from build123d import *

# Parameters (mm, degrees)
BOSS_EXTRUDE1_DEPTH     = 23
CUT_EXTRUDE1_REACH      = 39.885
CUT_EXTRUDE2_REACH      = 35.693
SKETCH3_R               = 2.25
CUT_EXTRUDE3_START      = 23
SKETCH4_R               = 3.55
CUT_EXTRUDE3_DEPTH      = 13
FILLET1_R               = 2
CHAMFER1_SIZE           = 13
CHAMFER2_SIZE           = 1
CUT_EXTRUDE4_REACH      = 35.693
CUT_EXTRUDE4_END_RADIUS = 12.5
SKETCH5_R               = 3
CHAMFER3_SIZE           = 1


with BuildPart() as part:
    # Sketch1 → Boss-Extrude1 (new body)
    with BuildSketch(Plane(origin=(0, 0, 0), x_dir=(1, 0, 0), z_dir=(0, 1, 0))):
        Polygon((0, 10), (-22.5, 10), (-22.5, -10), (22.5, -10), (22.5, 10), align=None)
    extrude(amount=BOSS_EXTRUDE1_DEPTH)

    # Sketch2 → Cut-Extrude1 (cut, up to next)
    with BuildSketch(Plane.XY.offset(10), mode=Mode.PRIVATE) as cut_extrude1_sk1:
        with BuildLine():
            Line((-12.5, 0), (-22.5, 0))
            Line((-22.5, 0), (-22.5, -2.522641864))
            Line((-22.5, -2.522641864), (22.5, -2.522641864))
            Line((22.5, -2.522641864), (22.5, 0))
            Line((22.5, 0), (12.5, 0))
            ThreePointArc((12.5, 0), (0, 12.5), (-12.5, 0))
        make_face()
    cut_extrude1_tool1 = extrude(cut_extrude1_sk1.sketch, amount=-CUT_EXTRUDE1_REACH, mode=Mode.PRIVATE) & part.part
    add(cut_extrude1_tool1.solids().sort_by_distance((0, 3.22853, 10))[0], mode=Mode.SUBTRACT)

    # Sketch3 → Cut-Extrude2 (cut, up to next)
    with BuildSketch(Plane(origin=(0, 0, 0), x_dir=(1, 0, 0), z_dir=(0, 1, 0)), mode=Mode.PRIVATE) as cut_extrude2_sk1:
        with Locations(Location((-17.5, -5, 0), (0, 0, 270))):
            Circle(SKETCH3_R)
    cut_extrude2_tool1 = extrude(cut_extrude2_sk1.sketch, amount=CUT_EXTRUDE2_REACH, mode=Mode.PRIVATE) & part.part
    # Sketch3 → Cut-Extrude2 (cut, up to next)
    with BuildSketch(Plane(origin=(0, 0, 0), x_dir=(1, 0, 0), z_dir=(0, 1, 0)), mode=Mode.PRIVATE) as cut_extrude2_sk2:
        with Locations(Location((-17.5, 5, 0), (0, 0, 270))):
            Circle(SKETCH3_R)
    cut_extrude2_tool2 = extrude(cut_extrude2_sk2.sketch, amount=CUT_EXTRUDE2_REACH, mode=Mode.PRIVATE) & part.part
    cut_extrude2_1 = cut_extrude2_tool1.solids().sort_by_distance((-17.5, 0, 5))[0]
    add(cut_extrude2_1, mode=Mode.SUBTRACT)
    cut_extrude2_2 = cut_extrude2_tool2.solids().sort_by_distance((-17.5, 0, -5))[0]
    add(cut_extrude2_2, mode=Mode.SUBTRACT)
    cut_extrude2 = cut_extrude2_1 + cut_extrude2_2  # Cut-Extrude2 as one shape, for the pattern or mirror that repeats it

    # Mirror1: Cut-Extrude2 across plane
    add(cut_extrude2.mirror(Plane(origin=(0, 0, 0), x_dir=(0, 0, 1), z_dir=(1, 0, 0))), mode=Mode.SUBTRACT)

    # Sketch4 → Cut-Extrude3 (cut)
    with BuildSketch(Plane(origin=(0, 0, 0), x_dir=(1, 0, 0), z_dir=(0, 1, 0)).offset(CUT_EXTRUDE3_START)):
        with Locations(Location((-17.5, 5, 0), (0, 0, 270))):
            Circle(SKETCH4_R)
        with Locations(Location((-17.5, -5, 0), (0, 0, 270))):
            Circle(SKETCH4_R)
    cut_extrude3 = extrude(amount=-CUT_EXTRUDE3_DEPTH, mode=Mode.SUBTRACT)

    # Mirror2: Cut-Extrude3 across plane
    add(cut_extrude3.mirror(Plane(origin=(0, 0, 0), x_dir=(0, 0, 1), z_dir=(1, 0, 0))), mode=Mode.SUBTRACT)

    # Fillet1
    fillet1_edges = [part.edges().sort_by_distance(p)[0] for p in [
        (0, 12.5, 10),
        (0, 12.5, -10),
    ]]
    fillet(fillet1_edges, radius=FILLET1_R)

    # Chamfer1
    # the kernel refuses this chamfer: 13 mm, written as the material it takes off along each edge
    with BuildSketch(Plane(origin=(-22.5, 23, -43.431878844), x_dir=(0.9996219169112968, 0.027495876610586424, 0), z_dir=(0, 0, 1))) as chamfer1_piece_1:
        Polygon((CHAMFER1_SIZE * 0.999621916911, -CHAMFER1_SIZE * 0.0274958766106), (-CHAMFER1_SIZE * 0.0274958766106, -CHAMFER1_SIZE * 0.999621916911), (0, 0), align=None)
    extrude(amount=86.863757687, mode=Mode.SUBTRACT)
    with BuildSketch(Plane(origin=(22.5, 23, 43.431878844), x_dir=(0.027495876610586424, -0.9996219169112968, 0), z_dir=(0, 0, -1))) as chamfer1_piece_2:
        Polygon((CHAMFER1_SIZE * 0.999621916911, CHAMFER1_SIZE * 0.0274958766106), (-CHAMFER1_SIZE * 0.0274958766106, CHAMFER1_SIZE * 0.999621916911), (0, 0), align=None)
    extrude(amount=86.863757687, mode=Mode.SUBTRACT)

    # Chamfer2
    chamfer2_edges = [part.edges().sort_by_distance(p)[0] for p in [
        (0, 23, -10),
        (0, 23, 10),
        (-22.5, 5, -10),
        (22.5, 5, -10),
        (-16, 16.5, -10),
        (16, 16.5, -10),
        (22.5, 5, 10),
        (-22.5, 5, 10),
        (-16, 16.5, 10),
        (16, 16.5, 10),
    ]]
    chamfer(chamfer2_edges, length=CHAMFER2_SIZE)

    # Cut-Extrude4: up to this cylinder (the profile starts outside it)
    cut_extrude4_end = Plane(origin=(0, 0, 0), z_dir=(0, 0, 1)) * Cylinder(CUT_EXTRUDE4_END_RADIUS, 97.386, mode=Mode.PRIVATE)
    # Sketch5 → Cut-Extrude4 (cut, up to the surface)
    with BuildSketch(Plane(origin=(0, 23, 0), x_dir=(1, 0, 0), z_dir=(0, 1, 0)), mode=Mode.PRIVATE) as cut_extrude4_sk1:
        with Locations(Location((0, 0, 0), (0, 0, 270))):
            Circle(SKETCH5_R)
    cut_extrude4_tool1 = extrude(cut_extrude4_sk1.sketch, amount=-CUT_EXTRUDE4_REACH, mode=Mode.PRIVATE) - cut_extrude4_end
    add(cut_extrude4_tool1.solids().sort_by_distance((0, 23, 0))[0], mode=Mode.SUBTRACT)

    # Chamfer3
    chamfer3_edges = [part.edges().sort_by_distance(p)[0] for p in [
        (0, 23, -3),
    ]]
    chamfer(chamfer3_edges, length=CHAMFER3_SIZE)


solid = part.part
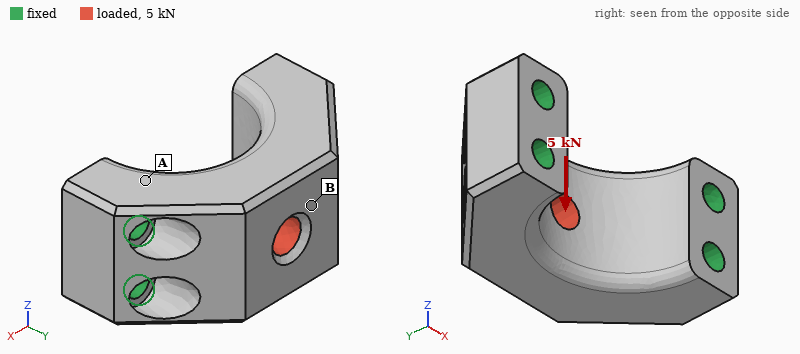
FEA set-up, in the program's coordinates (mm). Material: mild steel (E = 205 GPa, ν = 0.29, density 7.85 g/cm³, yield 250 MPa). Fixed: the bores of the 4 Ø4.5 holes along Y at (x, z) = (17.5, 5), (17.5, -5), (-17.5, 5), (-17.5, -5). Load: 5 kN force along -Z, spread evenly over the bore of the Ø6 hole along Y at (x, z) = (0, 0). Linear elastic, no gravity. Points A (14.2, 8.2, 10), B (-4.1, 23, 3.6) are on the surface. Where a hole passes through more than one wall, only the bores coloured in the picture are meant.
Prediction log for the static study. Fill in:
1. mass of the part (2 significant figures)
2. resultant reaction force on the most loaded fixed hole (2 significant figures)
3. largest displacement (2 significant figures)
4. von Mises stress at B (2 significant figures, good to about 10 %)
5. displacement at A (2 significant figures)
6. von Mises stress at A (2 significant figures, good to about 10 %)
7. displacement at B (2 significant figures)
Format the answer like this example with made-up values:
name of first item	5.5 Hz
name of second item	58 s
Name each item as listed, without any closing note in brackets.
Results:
mass of the part	83 g
resultant reaction force on the most loaded fixed hole	2.6 kN
largest displacement	8.7 µm
von Mises stress at B	18 MPa
displacement at A	1.9 µm
von Mises stress at A	55 MPa
displacement at B	7.9 µm
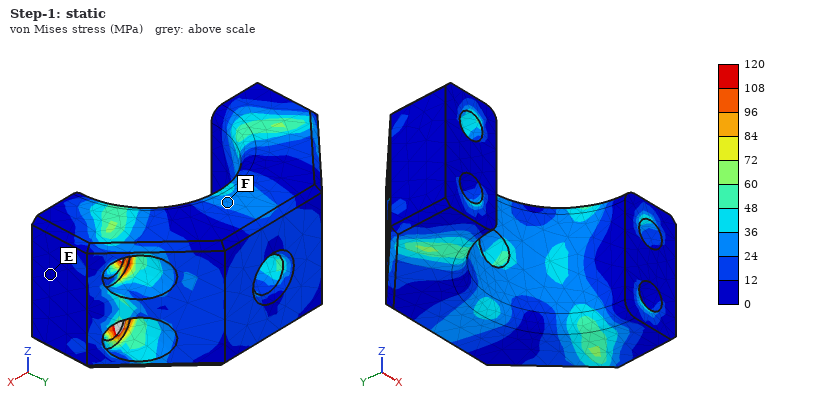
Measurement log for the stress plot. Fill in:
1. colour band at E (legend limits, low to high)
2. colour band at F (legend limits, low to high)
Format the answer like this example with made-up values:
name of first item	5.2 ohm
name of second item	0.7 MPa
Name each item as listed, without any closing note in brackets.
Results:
colour band at E	0 to 12 MPa
colour band at F	24 to 36 MPa
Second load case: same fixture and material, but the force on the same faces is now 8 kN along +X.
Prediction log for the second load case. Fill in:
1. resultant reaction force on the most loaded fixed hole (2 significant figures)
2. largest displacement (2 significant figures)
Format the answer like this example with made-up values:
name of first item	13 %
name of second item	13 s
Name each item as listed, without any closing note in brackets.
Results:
resultant reaction force on the most loaded fixed hole	2.3 kN
largest displacement	4.7 µm
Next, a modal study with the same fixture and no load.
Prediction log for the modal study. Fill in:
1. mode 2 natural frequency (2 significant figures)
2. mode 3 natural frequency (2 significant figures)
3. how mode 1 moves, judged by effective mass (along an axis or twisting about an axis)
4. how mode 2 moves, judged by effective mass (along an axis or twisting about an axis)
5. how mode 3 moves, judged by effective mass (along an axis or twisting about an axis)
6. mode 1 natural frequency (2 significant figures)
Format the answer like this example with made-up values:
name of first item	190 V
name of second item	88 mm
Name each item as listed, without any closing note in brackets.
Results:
mode 2 natural frequency	35 kHz
mode 3 natural frequency	37 kHz
how mode 1 moves, judged by effective mass	along Z
how mode 2 moves, judged by effective mass	along X
how mode 3 moves, judged by effective mass	twisting about Y
mode 1 natural frequency	21 kHz
